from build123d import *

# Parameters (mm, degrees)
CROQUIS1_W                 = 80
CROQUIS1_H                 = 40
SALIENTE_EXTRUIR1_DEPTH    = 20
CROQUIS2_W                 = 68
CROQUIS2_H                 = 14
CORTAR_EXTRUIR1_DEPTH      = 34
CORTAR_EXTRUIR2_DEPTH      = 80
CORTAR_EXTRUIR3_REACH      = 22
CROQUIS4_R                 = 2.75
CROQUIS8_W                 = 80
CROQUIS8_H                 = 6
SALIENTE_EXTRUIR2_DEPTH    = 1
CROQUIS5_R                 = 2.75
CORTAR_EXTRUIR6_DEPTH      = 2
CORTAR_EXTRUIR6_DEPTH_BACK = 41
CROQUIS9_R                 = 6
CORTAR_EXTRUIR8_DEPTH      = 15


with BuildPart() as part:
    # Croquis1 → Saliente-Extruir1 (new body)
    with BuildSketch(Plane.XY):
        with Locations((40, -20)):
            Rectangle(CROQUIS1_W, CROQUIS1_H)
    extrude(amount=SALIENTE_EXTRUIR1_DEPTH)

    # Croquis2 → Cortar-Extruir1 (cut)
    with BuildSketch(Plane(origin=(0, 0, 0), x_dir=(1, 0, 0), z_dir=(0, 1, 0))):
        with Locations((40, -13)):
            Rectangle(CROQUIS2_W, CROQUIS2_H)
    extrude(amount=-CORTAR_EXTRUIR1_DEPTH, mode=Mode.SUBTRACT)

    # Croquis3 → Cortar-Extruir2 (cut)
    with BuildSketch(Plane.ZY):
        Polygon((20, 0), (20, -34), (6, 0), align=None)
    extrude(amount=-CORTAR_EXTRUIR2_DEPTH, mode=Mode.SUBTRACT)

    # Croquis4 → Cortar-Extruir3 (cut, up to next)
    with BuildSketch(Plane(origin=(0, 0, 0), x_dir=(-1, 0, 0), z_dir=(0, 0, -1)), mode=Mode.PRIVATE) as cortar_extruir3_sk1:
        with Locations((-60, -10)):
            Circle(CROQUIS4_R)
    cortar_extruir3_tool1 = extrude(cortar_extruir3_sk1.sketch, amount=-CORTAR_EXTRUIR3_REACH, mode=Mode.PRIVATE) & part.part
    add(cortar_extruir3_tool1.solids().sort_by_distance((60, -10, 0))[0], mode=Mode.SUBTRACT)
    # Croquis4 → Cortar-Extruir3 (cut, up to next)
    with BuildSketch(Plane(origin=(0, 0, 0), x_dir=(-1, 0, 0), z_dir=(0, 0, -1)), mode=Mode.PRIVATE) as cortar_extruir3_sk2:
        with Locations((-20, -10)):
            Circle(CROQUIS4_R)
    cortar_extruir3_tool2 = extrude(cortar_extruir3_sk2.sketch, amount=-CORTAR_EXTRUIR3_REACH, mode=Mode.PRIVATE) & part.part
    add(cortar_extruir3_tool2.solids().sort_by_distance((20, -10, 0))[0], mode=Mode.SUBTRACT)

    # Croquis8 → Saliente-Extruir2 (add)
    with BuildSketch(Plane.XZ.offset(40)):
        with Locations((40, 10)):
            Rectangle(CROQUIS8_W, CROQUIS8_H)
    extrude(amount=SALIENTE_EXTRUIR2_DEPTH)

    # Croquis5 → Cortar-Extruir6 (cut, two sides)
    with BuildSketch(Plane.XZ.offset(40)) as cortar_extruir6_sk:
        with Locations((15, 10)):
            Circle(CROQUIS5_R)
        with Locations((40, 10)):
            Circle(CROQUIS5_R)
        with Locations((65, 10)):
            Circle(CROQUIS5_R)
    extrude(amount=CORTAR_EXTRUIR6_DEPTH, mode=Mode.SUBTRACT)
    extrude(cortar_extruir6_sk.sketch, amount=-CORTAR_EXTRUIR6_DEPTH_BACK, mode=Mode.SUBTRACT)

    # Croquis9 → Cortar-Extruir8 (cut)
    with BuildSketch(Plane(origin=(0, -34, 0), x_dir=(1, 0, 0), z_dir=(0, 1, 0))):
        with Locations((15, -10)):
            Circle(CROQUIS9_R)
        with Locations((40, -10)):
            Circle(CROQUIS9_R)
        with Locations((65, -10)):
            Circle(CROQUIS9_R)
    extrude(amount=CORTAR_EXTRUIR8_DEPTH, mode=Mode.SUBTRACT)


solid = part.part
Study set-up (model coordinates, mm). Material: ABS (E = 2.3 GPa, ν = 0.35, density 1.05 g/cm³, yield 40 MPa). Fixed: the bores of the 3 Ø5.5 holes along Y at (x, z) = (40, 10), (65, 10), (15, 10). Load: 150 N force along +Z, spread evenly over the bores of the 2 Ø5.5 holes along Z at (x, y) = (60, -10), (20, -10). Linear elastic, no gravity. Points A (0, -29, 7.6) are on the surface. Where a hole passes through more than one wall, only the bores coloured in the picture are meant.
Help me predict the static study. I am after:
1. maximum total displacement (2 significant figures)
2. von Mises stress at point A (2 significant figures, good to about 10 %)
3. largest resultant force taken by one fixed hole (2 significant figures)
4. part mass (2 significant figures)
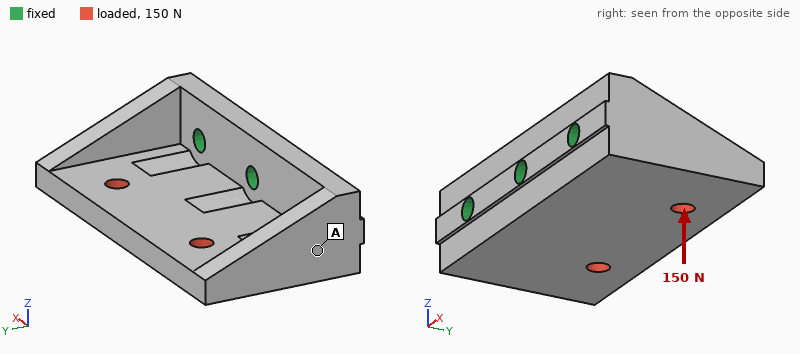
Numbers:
0.47 mm
1.6 MPa
57 N
29 g
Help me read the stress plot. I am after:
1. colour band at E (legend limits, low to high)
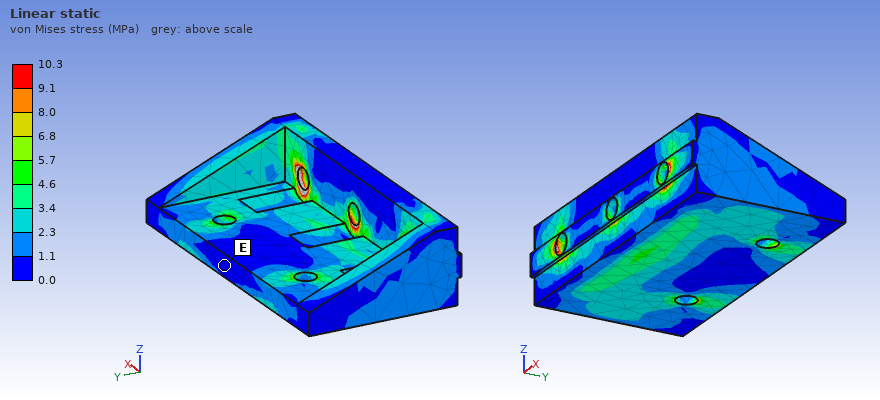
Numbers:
0.0 to 1.1 MPa
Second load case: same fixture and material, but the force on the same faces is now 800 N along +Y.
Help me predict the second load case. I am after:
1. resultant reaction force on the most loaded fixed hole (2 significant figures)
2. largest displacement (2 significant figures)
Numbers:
270 N
0.21 mm
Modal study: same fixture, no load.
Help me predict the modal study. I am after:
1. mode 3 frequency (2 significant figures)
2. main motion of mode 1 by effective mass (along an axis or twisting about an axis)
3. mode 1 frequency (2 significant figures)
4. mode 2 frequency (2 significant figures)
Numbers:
2600 Hz
along Z
1100 Hz
1500 Hz
